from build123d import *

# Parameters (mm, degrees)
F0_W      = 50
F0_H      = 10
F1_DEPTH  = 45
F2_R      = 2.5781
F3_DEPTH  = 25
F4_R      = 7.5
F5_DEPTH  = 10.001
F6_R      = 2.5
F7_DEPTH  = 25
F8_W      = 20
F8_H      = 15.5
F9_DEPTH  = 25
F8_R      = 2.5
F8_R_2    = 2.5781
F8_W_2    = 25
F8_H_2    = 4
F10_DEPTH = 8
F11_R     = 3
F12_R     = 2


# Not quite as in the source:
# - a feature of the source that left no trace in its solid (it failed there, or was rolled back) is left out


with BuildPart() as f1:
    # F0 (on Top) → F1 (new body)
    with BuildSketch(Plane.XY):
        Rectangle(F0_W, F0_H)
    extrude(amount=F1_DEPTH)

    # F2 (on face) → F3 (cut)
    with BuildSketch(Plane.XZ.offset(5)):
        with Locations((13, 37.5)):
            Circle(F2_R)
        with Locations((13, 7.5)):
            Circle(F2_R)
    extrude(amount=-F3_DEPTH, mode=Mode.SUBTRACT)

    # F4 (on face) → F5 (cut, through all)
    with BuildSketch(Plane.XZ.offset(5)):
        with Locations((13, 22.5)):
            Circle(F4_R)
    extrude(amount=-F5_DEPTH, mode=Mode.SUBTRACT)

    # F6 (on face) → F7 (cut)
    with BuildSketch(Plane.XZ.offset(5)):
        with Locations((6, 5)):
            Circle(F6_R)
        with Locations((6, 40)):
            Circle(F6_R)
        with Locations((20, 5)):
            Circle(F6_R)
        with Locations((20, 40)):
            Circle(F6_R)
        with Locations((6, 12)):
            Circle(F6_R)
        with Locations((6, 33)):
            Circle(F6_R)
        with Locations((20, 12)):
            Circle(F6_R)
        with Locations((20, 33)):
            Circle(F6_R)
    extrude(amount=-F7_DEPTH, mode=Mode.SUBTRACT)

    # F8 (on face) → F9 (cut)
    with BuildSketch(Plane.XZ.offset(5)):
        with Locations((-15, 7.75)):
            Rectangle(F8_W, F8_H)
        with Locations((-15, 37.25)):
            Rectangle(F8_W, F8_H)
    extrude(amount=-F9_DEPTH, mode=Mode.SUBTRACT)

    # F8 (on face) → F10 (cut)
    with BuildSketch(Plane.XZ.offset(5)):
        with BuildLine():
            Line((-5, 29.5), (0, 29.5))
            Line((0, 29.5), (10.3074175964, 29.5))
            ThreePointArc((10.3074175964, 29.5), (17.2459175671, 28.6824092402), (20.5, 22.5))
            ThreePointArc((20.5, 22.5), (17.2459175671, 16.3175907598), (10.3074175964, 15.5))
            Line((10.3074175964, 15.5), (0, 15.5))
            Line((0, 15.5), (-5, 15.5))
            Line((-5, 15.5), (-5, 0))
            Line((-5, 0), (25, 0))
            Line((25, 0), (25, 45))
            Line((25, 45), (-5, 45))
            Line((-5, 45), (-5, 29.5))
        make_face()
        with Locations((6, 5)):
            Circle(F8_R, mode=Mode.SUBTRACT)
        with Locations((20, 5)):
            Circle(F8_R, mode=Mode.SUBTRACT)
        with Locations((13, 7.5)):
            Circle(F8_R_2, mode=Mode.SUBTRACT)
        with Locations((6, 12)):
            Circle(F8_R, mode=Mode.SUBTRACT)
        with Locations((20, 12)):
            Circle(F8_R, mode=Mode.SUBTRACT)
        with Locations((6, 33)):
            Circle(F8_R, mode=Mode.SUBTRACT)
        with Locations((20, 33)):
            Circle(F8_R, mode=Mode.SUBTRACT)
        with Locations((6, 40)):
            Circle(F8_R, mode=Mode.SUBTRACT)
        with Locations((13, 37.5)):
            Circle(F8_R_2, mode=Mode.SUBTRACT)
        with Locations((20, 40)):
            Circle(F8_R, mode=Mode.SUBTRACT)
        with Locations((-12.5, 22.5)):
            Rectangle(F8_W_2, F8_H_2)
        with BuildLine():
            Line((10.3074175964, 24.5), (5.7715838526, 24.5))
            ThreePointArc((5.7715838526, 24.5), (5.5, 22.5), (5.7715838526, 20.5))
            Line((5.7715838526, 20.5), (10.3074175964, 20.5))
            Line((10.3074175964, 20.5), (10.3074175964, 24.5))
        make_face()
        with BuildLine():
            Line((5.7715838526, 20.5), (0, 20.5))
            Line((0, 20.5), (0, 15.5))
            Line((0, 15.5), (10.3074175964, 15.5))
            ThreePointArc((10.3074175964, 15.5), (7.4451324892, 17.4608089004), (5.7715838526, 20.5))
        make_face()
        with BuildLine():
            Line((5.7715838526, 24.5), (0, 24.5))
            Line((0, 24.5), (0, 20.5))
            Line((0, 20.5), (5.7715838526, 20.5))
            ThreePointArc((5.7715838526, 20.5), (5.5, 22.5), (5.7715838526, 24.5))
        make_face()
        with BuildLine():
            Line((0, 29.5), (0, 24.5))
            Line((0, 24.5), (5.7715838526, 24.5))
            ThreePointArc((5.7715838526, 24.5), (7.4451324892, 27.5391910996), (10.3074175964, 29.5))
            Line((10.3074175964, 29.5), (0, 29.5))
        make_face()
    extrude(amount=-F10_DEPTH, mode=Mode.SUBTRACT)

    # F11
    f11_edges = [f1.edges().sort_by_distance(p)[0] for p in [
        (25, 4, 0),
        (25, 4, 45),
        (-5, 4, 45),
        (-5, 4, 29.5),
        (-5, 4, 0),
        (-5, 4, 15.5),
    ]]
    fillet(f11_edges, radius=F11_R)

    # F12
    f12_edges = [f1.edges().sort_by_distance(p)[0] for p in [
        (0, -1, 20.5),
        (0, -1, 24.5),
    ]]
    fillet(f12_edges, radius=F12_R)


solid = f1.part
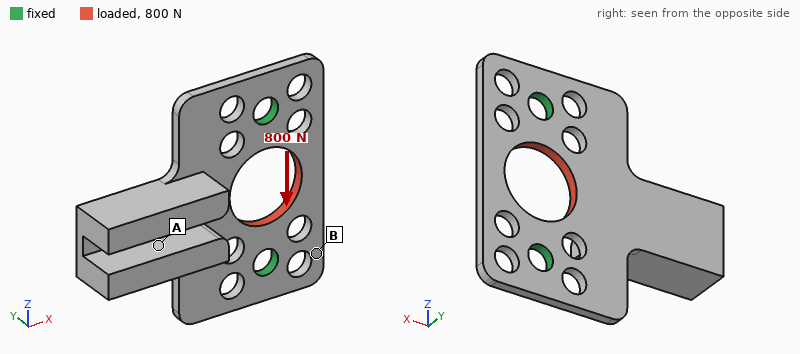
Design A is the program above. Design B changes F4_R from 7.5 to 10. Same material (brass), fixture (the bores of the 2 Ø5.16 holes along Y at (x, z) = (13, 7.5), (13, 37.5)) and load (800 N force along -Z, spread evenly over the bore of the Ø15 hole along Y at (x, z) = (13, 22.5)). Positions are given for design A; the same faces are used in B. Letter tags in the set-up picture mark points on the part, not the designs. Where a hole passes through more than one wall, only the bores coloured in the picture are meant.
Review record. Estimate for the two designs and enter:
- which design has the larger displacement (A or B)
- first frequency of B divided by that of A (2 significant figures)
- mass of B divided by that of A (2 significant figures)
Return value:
B
0.84
0.94
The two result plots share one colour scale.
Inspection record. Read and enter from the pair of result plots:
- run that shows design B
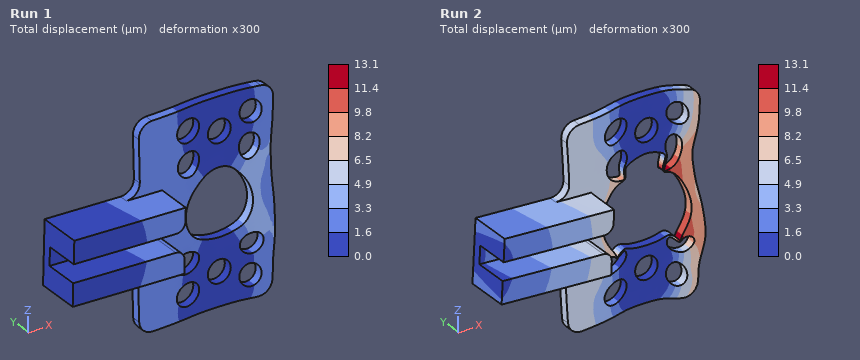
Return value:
Run 2
